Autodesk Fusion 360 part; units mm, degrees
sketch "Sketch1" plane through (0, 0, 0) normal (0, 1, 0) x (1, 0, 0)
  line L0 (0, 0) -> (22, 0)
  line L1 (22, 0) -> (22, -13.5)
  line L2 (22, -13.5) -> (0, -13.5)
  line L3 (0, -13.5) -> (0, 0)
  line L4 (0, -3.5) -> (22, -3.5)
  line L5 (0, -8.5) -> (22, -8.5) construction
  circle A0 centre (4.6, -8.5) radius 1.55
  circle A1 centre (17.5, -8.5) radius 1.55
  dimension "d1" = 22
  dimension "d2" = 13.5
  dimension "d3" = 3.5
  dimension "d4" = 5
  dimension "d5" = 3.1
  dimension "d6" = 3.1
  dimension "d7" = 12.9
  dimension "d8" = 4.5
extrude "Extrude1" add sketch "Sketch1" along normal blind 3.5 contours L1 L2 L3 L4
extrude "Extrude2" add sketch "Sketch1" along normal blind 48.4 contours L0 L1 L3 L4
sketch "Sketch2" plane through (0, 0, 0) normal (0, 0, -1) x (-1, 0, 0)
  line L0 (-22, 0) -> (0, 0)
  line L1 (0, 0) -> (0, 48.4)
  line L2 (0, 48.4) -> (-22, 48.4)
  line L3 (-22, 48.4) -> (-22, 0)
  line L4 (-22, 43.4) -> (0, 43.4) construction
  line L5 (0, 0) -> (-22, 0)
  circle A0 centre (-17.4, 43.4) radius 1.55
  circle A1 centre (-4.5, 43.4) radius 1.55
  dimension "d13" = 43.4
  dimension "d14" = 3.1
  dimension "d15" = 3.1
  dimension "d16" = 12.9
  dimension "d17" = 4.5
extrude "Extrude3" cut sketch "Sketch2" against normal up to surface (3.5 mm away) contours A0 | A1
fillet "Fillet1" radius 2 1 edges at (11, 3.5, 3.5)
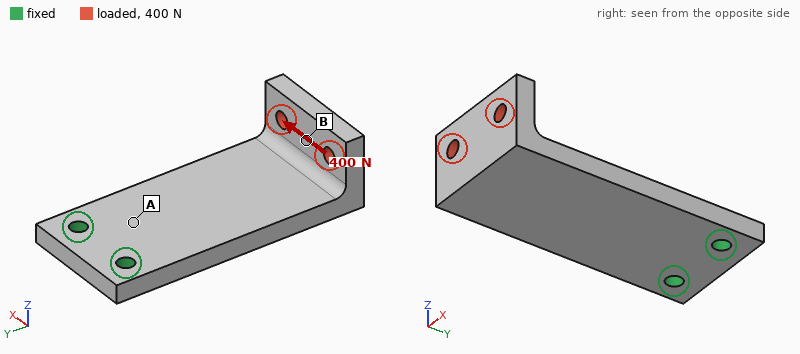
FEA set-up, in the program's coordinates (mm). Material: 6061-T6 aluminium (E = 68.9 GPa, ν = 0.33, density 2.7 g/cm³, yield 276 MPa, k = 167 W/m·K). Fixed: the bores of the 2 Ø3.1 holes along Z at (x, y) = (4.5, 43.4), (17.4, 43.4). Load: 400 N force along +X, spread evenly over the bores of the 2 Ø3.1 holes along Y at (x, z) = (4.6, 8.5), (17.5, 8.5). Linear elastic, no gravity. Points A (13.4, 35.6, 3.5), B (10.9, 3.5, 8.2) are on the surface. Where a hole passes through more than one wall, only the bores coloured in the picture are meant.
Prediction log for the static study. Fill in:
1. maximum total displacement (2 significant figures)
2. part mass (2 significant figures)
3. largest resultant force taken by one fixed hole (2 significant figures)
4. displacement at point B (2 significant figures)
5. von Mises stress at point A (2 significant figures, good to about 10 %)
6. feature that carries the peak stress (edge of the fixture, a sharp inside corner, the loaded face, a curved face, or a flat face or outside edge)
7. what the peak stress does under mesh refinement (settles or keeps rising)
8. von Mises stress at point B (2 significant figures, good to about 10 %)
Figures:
0.24 mm
12 g
1.2 kN
0.13 mm
59 MPa
edge of the fixture
keeps rising
19 MPa
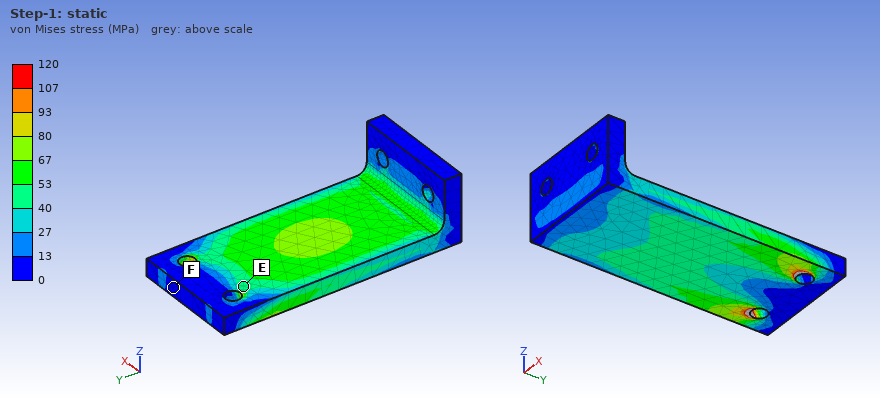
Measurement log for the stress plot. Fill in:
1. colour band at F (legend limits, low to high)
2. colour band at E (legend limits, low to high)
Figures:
0 to 13 MPa
40 to 53 MPa
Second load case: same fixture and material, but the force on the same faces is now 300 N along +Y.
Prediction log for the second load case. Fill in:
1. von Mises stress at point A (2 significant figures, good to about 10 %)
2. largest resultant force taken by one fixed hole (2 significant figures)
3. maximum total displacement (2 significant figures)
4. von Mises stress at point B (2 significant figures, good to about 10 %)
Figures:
45 MPa
150 N
0.38 mm
8.7 MPa
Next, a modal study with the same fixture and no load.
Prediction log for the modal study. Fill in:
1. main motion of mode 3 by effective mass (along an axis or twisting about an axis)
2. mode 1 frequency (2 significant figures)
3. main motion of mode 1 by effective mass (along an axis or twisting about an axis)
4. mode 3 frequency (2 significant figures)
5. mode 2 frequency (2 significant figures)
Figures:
along X
1100 Hz
along Z
6600 Hz
4000 Hz
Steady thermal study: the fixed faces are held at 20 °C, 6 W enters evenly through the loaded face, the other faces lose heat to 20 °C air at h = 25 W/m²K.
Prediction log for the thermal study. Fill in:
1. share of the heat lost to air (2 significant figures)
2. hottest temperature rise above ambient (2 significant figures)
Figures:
13 %
20 K
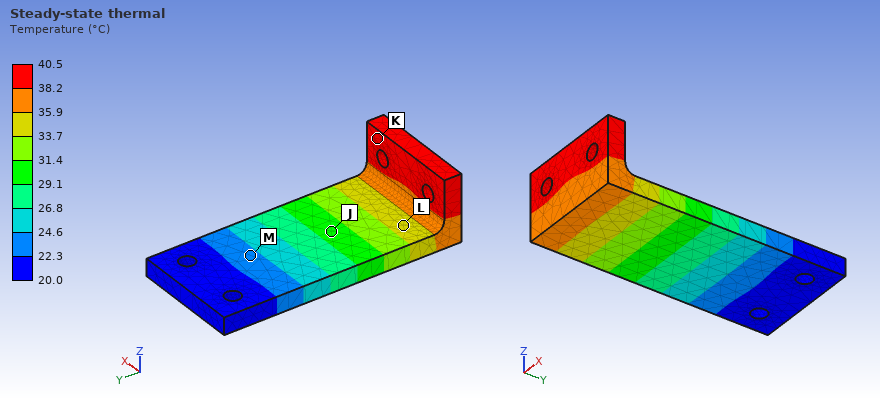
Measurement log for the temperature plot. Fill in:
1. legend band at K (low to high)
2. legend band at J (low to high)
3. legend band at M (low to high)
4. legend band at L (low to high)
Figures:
38.2 to 40.5 °C
29.1 to 31.4 °C
22.3 to 24.6 °C
33.7 to 35.9 °C
